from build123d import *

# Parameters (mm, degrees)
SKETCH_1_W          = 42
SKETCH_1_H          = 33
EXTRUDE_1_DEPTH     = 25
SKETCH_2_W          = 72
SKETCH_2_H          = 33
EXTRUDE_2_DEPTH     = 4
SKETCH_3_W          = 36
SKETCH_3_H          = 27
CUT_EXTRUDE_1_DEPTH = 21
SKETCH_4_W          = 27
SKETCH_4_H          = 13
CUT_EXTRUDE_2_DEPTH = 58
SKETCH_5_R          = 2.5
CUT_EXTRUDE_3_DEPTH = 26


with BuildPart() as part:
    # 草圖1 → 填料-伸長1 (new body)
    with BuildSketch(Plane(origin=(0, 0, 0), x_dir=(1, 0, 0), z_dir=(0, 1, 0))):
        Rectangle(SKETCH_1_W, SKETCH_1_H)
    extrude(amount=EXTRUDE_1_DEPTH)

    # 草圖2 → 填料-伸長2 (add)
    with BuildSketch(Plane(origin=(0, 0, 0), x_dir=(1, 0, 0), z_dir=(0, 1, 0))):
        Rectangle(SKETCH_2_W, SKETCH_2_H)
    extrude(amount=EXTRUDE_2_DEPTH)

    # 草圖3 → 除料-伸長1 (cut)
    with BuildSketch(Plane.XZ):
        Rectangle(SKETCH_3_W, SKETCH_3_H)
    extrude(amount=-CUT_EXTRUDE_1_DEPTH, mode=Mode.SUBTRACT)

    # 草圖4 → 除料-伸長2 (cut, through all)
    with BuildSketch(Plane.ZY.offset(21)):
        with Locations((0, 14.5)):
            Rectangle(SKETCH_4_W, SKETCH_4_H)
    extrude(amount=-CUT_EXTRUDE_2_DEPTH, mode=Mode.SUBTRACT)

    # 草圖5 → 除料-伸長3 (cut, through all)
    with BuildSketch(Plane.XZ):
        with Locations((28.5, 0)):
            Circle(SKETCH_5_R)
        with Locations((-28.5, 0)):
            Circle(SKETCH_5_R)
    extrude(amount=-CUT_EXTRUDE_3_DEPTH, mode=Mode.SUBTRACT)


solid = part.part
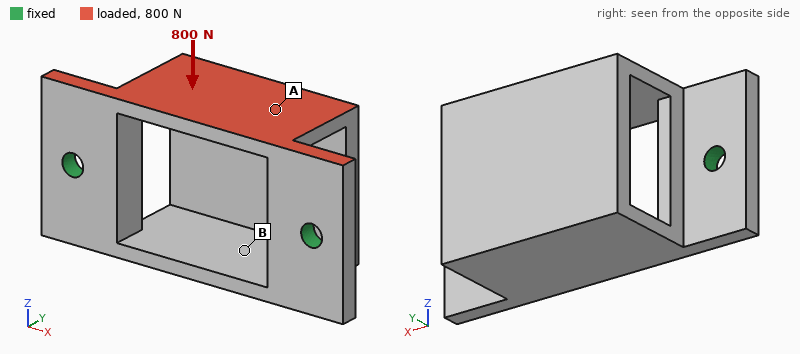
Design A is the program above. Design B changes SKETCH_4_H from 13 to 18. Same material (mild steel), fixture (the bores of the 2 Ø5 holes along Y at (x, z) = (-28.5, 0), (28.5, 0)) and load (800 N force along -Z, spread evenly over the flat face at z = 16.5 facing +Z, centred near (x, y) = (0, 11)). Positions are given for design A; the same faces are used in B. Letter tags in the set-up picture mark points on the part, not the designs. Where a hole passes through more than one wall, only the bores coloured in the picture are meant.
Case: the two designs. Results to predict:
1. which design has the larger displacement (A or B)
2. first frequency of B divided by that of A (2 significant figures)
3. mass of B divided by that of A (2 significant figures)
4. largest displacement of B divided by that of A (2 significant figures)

B
0.92
0.80
2.0
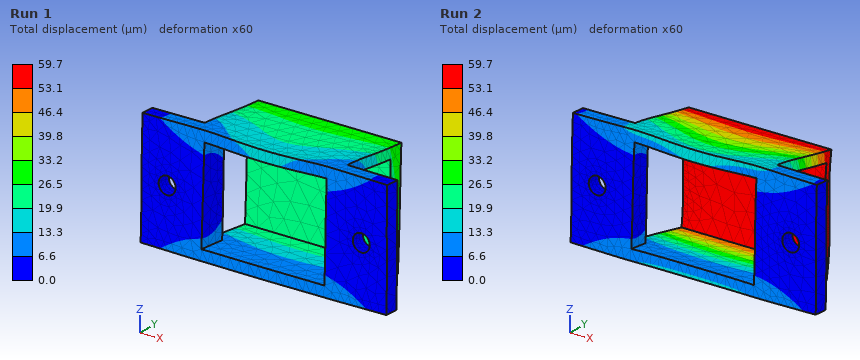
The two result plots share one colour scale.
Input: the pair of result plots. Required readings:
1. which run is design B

Run 2
